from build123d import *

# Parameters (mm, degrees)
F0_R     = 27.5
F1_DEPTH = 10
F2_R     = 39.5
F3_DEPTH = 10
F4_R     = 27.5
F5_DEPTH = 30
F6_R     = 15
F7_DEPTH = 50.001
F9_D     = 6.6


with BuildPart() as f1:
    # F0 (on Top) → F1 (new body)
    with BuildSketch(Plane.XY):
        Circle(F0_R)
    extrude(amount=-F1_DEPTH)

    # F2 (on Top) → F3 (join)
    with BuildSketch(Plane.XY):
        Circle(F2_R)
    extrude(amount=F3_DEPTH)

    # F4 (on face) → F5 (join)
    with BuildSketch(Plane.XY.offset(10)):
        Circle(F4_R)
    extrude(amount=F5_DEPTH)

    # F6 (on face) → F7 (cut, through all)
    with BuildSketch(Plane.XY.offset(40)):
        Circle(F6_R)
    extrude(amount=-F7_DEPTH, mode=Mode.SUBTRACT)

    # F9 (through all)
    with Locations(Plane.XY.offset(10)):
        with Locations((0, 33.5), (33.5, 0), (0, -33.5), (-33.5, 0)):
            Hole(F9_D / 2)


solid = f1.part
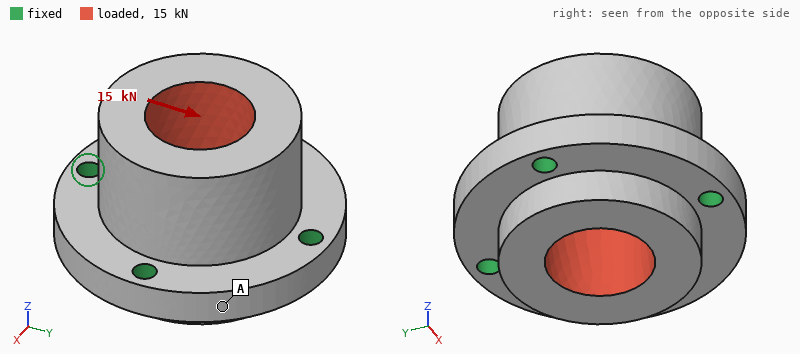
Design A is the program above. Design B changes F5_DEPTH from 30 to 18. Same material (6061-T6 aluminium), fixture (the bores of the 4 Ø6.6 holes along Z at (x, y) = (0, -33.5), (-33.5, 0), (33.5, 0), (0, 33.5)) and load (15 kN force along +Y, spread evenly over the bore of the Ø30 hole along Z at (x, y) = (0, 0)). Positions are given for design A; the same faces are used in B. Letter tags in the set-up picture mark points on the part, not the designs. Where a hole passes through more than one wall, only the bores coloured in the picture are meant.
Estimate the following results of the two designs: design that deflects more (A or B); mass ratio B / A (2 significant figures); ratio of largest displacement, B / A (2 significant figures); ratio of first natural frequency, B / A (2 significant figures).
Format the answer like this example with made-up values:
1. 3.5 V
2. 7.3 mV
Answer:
1. A
2. 0.81
3. 0.54
4. 1.4
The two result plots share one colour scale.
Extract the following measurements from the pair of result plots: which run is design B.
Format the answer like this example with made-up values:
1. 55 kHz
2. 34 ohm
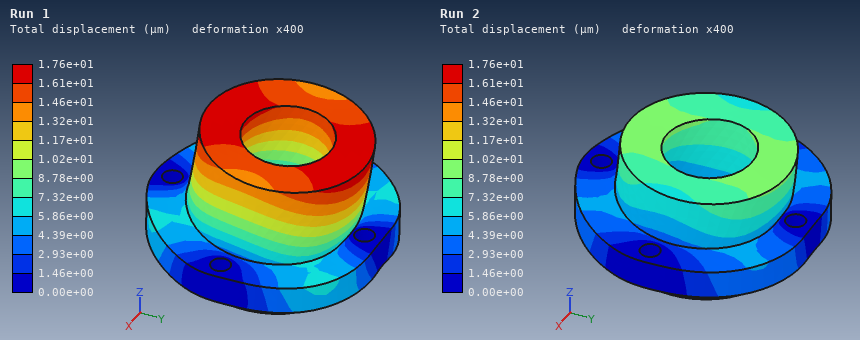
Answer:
1. Run 2
